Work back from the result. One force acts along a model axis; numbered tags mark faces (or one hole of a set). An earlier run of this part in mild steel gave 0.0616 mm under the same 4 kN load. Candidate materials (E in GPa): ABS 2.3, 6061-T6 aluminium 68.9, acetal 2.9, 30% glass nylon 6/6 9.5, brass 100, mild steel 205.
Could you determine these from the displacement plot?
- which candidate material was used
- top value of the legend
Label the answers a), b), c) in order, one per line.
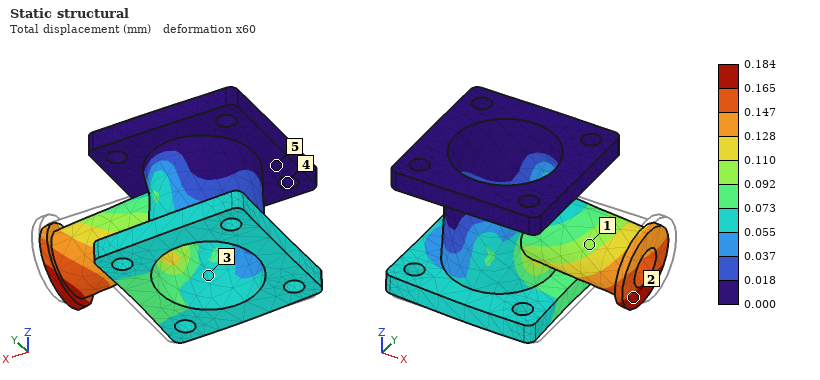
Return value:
a) 6061-T6 aluminium
b) 0.184 mm
